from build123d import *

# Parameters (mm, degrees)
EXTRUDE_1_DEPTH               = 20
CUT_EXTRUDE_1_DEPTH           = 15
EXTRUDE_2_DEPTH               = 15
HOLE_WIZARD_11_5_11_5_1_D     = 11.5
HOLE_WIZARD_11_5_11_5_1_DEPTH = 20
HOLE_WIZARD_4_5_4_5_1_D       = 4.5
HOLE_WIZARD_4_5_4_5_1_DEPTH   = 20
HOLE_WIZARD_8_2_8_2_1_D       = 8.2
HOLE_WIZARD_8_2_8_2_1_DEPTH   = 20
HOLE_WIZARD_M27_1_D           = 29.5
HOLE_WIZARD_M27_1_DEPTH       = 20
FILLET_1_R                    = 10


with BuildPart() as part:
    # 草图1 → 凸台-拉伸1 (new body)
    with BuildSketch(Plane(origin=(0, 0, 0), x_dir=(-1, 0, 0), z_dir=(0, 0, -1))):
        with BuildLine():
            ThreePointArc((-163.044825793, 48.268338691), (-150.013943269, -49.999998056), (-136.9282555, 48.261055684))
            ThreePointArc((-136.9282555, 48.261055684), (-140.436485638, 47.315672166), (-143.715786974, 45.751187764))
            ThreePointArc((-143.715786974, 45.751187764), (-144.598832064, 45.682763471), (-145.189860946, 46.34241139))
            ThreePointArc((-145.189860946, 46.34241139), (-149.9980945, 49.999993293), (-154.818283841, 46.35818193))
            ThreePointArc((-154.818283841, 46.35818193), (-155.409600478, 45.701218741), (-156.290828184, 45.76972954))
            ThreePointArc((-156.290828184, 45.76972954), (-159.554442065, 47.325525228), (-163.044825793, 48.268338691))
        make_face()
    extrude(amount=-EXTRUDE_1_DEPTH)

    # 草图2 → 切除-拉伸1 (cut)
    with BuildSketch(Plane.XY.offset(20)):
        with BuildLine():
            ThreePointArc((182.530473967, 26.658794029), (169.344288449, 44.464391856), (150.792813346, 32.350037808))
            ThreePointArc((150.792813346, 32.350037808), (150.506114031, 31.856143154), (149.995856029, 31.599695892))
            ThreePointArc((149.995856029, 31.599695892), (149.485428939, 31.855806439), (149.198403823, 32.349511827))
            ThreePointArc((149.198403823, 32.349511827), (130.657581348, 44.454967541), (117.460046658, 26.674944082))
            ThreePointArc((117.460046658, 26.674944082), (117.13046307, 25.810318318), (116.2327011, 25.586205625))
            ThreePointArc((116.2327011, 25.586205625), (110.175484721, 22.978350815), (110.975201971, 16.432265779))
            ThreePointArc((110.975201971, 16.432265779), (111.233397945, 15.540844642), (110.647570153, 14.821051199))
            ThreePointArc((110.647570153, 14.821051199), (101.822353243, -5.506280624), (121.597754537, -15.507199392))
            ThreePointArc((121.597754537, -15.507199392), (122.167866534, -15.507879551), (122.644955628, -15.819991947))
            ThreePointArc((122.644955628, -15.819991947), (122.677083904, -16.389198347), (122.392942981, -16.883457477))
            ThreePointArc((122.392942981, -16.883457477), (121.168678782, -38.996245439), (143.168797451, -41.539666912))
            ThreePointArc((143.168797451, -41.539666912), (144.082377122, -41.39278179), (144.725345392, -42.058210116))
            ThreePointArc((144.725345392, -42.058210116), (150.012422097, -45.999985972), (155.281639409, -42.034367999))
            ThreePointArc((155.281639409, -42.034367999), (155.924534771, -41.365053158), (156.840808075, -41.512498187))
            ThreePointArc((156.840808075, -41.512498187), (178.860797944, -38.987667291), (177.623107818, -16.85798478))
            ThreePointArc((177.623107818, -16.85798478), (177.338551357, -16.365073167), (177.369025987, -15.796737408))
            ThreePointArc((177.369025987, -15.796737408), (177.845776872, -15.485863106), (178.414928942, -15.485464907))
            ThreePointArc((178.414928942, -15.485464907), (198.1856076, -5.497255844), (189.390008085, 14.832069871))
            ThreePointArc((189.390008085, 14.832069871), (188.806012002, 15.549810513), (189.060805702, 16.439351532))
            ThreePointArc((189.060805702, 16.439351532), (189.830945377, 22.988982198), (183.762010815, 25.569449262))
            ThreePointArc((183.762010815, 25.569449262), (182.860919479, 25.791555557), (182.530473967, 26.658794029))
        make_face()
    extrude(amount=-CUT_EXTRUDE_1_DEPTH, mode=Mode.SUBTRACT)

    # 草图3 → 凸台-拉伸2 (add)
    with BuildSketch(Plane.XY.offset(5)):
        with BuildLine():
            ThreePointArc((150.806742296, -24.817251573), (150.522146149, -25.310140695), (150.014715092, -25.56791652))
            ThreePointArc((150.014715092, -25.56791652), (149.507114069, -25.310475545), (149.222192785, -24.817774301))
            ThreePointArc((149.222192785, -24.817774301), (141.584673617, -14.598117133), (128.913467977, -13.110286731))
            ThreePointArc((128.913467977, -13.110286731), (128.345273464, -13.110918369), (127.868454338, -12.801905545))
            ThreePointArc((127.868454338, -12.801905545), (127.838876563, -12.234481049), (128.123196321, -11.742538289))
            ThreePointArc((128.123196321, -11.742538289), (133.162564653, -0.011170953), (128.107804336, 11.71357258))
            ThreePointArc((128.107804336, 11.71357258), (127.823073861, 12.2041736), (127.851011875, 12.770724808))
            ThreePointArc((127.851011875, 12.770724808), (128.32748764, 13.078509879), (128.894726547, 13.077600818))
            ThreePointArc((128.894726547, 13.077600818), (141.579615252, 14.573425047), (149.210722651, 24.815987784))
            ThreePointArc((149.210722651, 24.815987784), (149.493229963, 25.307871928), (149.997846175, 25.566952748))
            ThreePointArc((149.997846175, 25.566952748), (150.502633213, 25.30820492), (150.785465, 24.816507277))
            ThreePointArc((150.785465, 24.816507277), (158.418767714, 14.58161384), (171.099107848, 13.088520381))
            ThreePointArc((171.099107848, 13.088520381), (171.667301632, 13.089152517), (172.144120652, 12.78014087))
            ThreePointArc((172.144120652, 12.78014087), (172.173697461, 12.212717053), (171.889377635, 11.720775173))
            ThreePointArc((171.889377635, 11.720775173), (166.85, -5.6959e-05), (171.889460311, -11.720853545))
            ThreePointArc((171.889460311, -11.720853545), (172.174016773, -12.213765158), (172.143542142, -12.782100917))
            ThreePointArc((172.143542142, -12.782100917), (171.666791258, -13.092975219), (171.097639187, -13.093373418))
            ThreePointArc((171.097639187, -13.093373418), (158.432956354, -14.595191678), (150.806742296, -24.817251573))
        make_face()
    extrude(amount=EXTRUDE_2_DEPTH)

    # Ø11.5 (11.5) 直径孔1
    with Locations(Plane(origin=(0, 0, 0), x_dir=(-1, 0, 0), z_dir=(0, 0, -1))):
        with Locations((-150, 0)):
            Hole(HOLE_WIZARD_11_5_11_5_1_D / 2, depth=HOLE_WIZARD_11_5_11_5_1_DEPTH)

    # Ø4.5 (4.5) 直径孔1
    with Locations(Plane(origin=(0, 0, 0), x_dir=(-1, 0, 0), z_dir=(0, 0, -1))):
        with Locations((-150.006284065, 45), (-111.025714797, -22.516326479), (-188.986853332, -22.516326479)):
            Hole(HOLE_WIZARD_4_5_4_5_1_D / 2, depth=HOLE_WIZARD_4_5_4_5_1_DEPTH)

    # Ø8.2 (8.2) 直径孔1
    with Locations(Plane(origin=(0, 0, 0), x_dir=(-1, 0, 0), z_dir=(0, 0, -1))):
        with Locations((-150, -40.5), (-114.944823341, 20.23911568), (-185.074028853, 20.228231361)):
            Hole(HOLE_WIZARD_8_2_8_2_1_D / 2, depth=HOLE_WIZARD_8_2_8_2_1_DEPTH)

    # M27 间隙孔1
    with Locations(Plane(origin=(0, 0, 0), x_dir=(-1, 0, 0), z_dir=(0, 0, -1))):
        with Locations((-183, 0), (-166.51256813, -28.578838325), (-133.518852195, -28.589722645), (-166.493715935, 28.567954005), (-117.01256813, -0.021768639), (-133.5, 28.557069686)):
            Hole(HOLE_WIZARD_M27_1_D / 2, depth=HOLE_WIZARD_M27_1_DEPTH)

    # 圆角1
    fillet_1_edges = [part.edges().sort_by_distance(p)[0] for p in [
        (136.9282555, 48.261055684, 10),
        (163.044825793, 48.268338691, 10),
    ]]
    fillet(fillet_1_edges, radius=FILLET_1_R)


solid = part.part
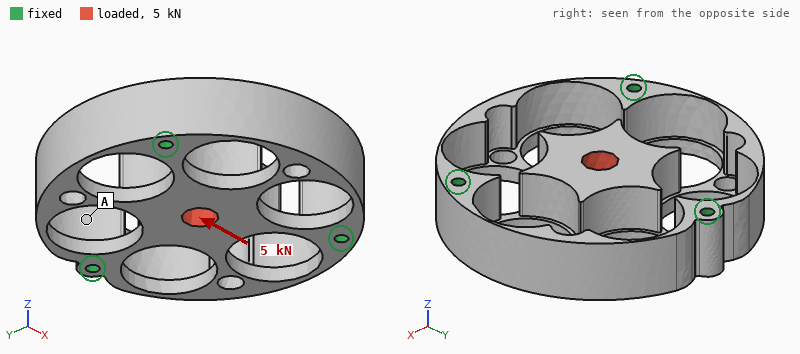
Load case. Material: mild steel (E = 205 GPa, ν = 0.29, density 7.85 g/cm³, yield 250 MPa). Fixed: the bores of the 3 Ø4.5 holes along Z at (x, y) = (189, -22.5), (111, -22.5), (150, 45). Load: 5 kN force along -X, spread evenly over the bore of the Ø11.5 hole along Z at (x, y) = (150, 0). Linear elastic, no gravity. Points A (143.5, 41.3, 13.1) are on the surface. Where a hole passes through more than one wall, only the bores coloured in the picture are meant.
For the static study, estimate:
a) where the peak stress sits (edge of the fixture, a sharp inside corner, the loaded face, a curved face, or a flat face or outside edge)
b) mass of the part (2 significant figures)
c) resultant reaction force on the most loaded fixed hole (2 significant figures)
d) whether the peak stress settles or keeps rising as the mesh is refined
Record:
a sharp inside corner
420 g
2.4 kN
keeps rising
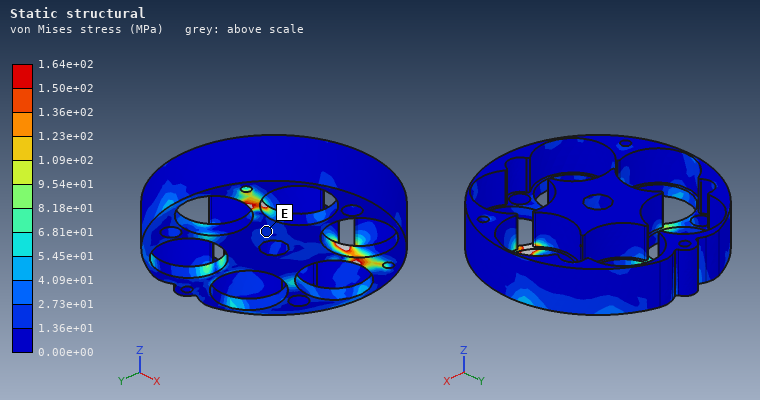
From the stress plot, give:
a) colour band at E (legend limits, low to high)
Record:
1.36e+01 to 2.73e+01 MPa
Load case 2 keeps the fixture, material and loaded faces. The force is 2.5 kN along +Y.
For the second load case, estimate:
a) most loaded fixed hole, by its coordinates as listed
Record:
(150, 45)
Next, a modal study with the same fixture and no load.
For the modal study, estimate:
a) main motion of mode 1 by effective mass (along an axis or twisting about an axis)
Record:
along Z
